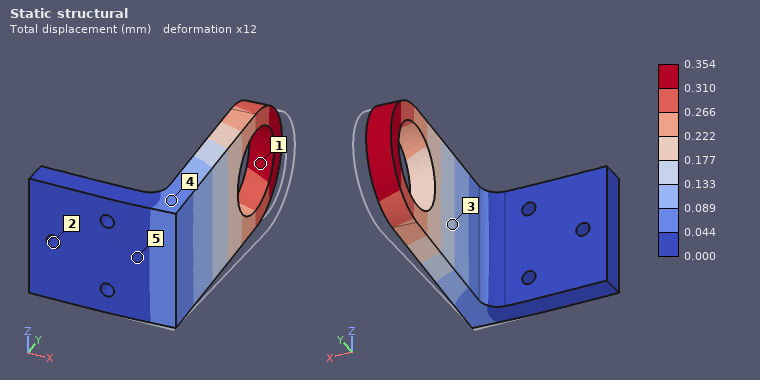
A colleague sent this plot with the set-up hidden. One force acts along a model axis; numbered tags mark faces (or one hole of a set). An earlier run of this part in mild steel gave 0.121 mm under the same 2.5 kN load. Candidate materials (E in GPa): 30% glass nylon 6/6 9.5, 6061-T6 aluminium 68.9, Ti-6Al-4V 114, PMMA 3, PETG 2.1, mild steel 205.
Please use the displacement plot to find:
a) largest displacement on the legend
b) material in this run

0.354 mm
6061-T6 aluminium
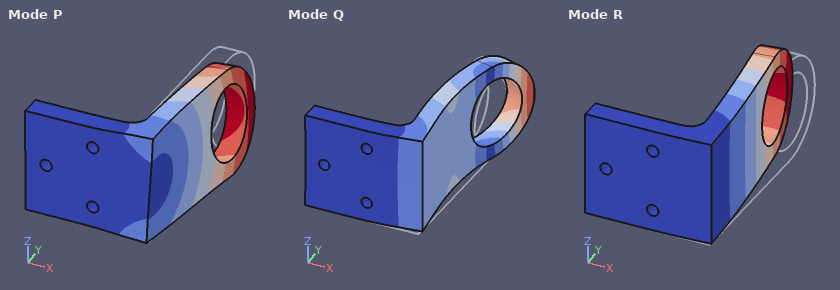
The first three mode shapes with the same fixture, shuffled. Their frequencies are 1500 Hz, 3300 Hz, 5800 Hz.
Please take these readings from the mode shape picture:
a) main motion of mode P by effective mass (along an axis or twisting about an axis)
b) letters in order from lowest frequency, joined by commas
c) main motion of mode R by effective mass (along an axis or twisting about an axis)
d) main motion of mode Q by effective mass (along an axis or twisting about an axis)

along Z
R, P, Q
along X
along Y
